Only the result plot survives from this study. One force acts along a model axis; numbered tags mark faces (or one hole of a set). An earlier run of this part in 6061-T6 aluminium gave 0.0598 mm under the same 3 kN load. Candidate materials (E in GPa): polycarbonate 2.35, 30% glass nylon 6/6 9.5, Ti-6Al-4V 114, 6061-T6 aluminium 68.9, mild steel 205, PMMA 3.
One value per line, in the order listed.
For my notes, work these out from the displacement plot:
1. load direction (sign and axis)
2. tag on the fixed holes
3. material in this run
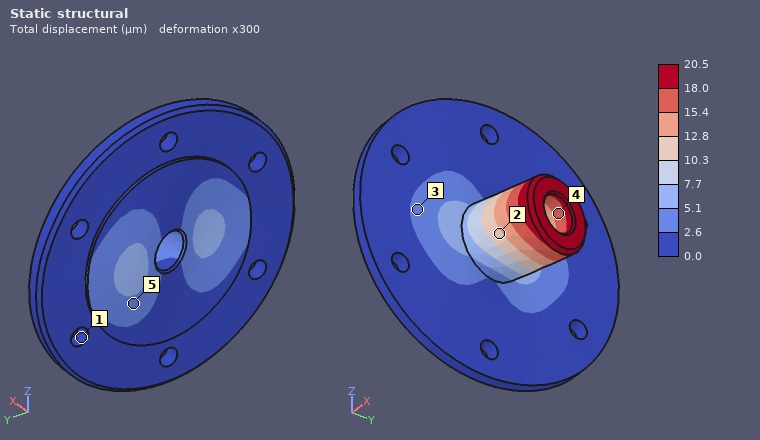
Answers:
+Y
1
mild steel
